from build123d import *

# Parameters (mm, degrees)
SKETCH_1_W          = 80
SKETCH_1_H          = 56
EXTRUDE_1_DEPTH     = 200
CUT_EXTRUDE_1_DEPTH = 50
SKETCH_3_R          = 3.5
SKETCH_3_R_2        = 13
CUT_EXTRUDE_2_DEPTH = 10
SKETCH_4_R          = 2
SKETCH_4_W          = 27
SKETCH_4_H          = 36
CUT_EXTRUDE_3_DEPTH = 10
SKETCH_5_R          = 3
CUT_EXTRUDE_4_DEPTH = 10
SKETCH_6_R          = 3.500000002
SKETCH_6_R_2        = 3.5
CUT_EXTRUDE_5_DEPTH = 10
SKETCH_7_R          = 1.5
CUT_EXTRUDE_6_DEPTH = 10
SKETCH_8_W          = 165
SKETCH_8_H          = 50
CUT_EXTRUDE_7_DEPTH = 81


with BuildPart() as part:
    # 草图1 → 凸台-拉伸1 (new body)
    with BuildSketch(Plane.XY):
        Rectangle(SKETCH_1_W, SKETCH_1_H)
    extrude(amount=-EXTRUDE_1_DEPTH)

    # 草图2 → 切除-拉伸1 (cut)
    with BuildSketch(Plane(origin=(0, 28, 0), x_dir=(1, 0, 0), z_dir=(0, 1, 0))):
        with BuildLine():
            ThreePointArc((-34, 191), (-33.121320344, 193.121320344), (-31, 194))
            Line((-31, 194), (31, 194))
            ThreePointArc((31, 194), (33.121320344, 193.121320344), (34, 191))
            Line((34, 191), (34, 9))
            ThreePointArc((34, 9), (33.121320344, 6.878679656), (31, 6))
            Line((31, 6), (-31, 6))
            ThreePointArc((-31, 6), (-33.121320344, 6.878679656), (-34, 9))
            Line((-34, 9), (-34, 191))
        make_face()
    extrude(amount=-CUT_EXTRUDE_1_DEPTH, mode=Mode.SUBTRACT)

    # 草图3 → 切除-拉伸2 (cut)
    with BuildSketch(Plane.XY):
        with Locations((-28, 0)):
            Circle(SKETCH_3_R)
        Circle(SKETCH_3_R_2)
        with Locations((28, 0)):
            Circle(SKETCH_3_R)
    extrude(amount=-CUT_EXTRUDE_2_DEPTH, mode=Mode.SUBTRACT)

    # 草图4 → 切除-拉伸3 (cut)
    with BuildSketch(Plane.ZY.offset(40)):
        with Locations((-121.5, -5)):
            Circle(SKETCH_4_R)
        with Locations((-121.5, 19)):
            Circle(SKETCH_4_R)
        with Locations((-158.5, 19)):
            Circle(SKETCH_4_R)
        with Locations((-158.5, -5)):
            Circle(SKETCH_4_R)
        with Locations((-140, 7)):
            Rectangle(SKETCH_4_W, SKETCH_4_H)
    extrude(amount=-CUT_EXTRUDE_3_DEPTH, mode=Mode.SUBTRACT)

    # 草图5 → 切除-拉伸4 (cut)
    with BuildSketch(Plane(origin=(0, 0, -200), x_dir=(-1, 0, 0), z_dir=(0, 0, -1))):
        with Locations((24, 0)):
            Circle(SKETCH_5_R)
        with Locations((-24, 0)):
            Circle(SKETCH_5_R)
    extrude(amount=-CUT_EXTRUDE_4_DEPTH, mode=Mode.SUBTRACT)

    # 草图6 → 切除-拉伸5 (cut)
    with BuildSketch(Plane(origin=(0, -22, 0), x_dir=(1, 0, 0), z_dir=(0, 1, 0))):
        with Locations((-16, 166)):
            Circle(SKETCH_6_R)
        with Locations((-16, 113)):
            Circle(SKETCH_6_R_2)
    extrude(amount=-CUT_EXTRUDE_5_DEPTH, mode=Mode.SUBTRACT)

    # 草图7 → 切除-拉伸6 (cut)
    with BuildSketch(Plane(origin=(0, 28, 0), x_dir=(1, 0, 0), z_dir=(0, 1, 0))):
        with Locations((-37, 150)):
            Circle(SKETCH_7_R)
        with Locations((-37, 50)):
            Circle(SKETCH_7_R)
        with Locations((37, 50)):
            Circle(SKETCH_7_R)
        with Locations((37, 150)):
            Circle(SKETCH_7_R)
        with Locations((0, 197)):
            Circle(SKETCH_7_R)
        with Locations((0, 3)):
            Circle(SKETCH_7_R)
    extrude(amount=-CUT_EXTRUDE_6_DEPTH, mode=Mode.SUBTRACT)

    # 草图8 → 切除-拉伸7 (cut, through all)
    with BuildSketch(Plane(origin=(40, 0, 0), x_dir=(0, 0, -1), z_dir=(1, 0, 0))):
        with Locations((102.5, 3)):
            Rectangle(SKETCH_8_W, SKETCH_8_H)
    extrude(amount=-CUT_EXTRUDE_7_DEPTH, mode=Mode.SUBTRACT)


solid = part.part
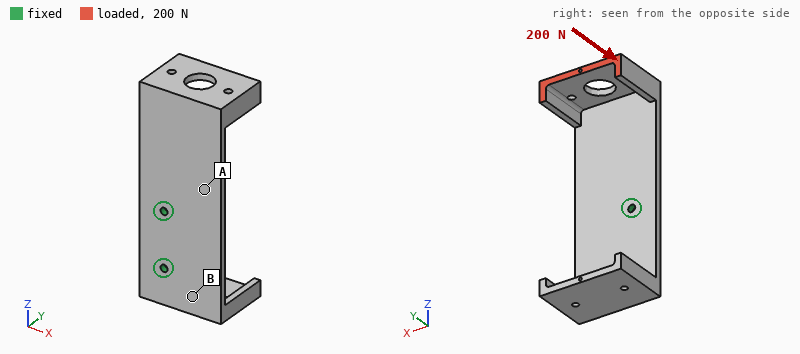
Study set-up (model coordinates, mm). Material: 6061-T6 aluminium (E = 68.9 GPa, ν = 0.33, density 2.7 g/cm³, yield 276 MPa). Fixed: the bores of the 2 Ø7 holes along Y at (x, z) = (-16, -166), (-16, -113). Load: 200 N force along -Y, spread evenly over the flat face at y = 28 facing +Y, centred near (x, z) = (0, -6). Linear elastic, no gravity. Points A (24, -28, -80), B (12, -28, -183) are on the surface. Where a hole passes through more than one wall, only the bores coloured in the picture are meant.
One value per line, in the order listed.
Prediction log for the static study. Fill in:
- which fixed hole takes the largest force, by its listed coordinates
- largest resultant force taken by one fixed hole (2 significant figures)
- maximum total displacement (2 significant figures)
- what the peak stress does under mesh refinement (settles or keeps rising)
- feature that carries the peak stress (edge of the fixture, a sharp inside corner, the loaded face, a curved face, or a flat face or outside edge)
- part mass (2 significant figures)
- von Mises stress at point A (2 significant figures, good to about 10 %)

(-16, -113)
370 N
1.2 mm
keeps rising
edge of the fixture
410 g
28 MPa
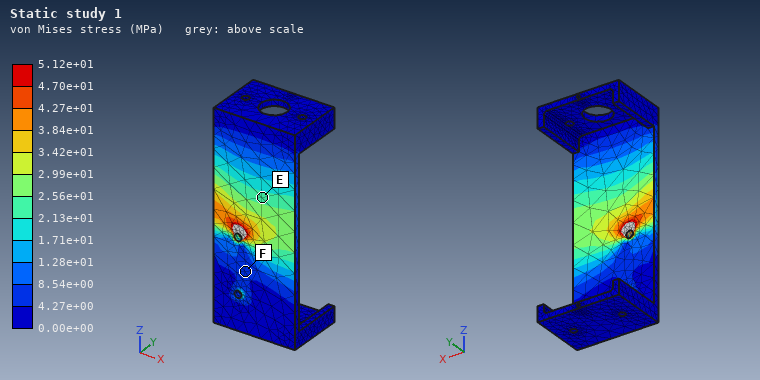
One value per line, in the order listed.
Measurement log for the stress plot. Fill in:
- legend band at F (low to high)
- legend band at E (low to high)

4.27e+00 to 8.54e+00 MPa
2.13e+01 to 2.56e+01 MPa
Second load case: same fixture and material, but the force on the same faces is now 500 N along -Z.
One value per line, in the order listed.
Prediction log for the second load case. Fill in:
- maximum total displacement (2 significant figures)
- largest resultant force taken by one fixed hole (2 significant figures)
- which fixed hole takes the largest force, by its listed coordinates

2.4 mm
440 N
(-16, -113)
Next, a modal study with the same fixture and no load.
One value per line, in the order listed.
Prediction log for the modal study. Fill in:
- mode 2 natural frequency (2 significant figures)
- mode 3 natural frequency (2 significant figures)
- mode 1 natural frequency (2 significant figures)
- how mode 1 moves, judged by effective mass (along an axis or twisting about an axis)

450 Hz
770 Hz
200 Hz
along Y
